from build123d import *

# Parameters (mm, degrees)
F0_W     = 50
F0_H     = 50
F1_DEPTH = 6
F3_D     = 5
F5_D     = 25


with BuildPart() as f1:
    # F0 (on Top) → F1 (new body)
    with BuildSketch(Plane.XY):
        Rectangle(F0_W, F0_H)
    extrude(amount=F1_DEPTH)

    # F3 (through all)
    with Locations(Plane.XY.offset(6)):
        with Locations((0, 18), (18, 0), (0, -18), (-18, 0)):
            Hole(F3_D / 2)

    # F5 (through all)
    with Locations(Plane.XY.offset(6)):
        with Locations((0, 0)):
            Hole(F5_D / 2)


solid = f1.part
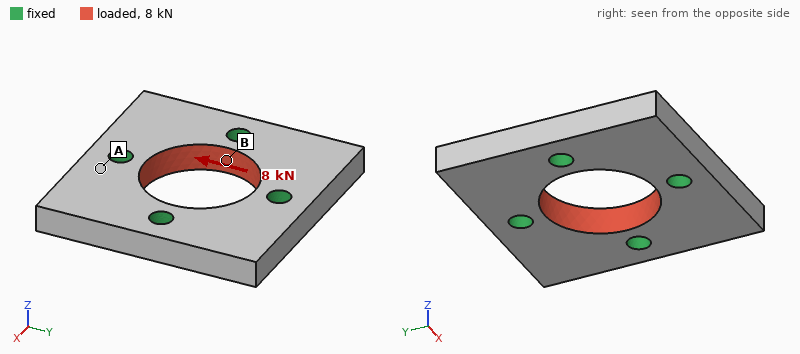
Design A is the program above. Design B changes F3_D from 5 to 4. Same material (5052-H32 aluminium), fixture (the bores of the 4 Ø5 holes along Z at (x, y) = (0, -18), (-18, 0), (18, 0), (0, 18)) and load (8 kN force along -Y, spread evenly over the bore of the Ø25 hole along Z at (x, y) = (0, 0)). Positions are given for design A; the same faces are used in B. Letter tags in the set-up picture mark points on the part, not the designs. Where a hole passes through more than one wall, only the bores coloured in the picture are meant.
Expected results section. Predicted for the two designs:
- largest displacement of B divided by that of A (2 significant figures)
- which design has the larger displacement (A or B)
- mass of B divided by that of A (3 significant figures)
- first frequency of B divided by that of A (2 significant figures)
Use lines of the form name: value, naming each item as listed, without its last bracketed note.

largest displacement of B divided by that of A: 1.1
which design has the larger displacement: B
mass of B divided by that of A: 1.01
first frequency of B divided by that of A: 0.93
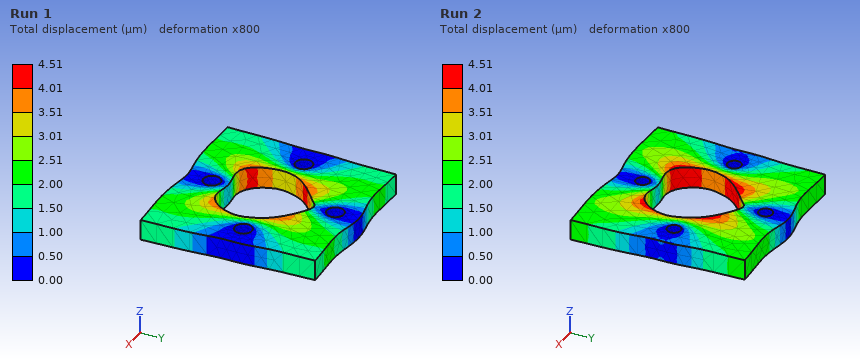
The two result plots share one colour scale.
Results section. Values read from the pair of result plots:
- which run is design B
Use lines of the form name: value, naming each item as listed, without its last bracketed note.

which run is design B: Run 2
